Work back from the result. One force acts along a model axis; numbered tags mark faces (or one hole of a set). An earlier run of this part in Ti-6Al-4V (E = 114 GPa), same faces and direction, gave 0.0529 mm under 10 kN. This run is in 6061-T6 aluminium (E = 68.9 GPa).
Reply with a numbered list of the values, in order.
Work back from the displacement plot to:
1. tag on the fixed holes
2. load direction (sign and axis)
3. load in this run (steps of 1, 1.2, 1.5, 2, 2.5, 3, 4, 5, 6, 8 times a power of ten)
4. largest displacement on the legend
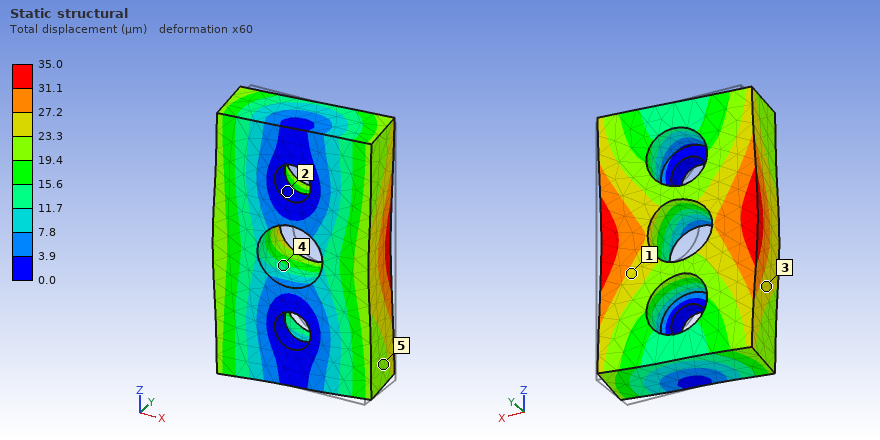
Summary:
1. 2
2. -X
3. 4 kN
4. 35.0 µm
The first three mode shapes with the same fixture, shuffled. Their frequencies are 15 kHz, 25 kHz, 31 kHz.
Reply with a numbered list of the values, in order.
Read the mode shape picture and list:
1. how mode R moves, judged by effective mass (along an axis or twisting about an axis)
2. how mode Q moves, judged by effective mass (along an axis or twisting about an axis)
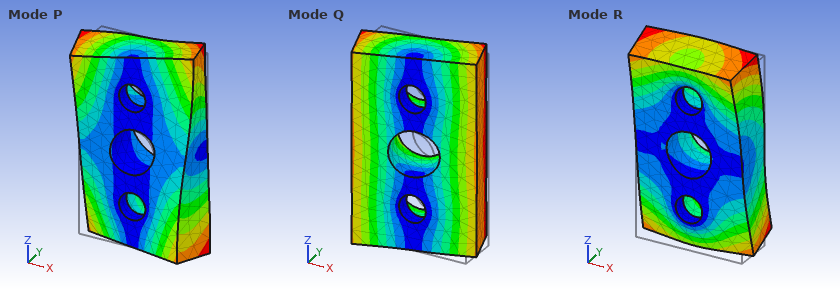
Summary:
1. along Z
2. along X
